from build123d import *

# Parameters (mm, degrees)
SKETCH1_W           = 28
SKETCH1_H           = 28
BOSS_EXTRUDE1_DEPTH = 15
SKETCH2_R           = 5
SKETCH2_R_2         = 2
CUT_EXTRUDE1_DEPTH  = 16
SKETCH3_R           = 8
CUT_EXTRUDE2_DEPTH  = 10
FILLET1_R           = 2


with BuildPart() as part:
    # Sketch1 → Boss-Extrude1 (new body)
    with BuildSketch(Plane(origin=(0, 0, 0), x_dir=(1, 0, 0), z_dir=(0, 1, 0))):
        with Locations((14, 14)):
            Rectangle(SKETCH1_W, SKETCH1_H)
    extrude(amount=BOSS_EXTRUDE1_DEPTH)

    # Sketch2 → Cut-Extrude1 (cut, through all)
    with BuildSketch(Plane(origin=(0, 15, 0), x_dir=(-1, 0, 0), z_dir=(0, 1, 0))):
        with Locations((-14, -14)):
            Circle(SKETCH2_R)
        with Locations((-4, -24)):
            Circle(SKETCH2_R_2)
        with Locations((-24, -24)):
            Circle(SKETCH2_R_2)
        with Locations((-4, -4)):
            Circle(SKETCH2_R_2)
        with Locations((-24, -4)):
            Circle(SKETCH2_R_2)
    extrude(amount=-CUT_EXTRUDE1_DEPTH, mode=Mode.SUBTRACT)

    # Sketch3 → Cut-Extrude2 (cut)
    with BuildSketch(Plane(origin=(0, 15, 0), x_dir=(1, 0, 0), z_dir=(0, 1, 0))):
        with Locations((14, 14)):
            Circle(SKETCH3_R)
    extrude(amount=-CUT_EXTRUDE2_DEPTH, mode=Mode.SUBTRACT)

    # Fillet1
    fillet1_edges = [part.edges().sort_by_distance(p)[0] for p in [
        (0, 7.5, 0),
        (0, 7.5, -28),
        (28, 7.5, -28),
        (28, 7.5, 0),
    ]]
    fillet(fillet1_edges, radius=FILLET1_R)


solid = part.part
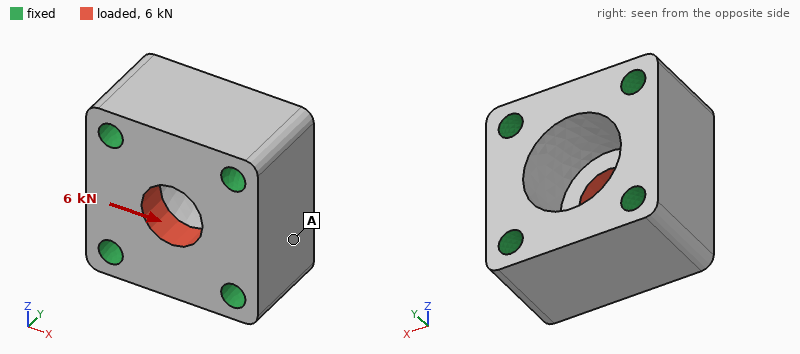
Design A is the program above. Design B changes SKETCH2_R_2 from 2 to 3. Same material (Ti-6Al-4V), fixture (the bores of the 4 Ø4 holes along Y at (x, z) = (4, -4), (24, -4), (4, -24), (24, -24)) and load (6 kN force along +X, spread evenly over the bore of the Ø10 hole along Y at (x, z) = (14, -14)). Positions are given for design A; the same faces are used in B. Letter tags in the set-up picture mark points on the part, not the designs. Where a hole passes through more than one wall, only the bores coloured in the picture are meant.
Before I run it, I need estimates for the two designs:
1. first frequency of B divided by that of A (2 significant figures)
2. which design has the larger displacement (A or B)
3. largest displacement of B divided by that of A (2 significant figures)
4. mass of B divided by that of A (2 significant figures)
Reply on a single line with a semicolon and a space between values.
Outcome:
1.3; A; 0.87; 0.89
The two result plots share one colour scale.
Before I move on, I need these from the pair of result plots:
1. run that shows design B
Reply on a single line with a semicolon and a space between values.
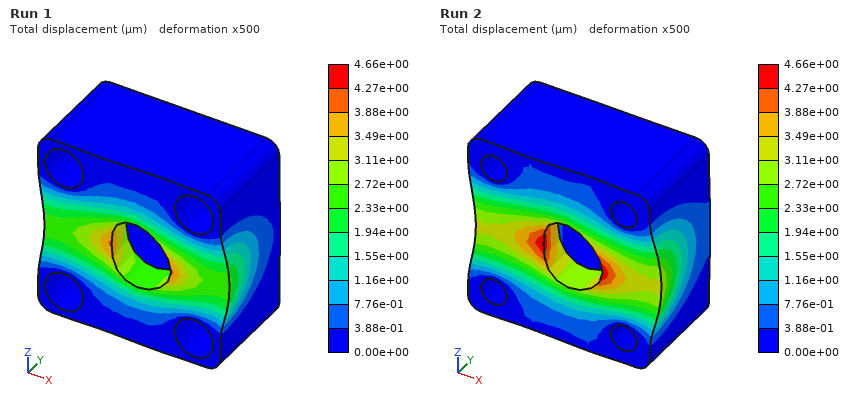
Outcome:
Run 1
